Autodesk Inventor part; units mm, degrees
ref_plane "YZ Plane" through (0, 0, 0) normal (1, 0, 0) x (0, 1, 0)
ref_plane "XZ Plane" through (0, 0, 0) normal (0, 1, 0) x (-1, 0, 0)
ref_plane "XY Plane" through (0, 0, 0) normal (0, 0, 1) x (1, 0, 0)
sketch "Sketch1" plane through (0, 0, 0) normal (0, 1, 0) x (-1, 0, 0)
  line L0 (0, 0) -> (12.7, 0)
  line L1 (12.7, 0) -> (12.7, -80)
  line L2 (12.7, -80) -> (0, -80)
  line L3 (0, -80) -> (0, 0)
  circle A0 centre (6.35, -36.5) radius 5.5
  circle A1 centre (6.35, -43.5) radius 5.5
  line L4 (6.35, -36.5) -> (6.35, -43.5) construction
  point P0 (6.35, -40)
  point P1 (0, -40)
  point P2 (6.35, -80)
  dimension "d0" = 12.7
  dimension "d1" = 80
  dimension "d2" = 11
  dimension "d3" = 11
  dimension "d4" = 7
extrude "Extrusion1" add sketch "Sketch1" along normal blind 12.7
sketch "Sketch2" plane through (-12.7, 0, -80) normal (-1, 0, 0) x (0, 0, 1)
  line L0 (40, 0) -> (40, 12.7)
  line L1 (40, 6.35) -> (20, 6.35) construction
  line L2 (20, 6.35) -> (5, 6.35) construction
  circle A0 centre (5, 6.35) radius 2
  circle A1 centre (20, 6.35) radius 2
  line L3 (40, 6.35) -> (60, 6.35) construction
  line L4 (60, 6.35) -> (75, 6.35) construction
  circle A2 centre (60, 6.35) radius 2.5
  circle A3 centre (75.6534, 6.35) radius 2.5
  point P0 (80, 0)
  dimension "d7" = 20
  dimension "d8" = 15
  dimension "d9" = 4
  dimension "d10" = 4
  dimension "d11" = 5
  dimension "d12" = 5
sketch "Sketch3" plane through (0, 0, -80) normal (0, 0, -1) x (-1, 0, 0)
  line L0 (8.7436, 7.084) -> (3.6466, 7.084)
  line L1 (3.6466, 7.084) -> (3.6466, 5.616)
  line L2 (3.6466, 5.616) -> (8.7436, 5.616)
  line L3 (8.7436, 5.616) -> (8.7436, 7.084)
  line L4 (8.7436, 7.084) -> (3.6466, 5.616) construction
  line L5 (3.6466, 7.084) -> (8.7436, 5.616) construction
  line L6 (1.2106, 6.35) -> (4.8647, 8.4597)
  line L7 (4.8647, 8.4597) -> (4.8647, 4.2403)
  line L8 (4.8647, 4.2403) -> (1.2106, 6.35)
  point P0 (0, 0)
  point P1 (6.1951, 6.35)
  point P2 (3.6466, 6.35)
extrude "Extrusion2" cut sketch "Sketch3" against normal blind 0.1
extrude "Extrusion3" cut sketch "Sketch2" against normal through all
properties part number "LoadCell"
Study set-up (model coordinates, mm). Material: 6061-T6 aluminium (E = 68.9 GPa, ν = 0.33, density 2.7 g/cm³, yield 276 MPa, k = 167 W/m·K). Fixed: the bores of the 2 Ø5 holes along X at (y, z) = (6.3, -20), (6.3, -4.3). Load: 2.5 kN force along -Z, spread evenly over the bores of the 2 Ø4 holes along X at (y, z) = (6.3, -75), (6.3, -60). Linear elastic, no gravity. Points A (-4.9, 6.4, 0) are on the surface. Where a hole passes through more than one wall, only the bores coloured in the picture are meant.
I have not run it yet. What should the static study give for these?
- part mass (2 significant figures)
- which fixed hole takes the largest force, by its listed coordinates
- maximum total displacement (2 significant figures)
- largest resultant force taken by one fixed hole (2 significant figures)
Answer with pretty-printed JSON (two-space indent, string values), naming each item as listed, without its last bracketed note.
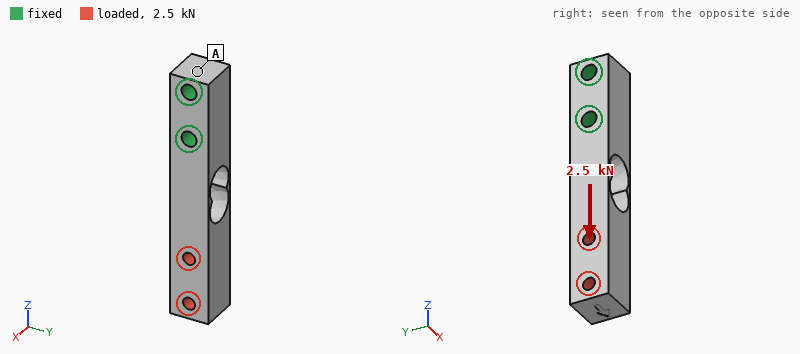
{
  "part mass": "27 g",
  "which fixed hole takes the largest force, by its listed coordinates": "(6.3, -20)",
  "maximum total displacement": "36 µm",
  "largest resultant force taken by one fixed hole": "2.3 kN"
}
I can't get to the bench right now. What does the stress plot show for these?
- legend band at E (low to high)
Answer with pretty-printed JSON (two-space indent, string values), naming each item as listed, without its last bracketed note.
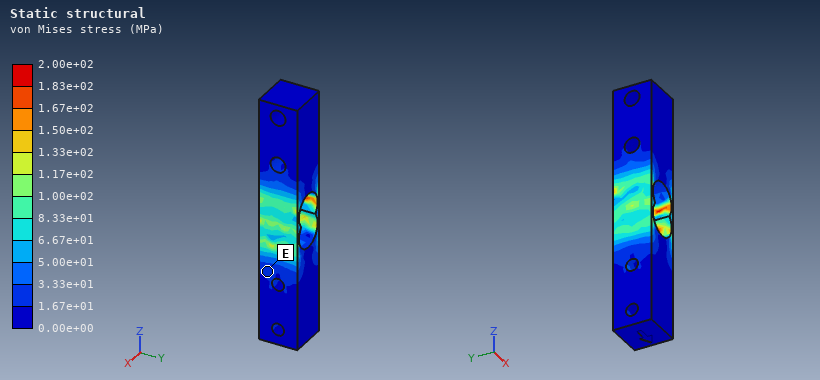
{
  "legend band at E": "1.67e+01 to 3.33e+01 MPa"
}
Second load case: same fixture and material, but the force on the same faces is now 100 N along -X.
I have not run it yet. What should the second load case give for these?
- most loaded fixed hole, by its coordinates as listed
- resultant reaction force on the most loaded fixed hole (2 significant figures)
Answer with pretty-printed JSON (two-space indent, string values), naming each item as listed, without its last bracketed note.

{
  "most loaded fixed hole, by its coordinates as listed": "(6.3, -20)",
  "resultant reaction force on the most loaded fixed hole": "130 N"
}
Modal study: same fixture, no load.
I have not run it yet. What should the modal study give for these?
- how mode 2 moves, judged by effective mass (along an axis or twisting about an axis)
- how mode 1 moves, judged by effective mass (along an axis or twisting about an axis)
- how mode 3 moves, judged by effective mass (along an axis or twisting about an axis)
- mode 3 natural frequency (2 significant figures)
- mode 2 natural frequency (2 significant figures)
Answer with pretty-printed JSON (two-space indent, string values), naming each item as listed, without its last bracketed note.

{
  "how mode 2 moves, judged by effective mass": "along Y",
  "how mode 1 moves, judged by effective mass": "along X",
  "how mode 3 moves, judged by effective mass": "twisting about Z",
  "mode 3 natural frequency": "6200 Hz",
  "mode 2 natural frequency": "1600 Hz"
}
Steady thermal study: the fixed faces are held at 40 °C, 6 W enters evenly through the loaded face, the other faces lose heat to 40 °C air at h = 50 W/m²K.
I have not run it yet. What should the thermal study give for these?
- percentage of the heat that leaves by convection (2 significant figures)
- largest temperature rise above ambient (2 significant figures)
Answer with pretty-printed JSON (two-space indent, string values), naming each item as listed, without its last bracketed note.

{
  "percentage of the heat that leaves by convection": "34 %",
  "largest temperature rise above ambient": "19 K"
}
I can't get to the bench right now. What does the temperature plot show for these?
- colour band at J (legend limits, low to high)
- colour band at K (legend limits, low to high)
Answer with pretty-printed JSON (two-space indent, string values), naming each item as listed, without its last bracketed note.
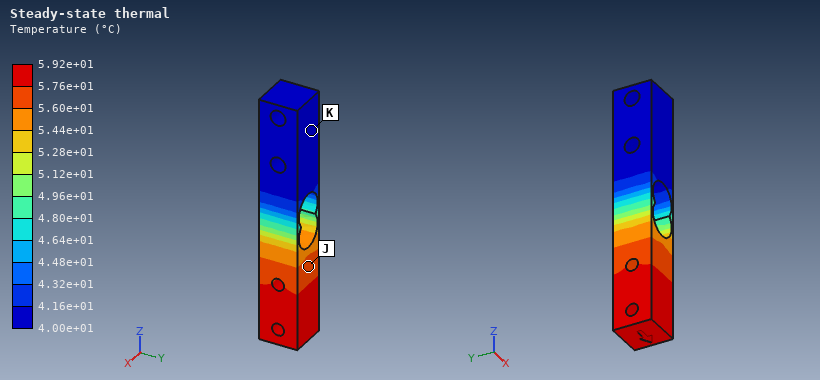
{
  "colour band at J": "5.60e+01 to 5.76e+01 °C",
  "colour band at K": "4.00e+01 to 4.16e+01 °C"
}
